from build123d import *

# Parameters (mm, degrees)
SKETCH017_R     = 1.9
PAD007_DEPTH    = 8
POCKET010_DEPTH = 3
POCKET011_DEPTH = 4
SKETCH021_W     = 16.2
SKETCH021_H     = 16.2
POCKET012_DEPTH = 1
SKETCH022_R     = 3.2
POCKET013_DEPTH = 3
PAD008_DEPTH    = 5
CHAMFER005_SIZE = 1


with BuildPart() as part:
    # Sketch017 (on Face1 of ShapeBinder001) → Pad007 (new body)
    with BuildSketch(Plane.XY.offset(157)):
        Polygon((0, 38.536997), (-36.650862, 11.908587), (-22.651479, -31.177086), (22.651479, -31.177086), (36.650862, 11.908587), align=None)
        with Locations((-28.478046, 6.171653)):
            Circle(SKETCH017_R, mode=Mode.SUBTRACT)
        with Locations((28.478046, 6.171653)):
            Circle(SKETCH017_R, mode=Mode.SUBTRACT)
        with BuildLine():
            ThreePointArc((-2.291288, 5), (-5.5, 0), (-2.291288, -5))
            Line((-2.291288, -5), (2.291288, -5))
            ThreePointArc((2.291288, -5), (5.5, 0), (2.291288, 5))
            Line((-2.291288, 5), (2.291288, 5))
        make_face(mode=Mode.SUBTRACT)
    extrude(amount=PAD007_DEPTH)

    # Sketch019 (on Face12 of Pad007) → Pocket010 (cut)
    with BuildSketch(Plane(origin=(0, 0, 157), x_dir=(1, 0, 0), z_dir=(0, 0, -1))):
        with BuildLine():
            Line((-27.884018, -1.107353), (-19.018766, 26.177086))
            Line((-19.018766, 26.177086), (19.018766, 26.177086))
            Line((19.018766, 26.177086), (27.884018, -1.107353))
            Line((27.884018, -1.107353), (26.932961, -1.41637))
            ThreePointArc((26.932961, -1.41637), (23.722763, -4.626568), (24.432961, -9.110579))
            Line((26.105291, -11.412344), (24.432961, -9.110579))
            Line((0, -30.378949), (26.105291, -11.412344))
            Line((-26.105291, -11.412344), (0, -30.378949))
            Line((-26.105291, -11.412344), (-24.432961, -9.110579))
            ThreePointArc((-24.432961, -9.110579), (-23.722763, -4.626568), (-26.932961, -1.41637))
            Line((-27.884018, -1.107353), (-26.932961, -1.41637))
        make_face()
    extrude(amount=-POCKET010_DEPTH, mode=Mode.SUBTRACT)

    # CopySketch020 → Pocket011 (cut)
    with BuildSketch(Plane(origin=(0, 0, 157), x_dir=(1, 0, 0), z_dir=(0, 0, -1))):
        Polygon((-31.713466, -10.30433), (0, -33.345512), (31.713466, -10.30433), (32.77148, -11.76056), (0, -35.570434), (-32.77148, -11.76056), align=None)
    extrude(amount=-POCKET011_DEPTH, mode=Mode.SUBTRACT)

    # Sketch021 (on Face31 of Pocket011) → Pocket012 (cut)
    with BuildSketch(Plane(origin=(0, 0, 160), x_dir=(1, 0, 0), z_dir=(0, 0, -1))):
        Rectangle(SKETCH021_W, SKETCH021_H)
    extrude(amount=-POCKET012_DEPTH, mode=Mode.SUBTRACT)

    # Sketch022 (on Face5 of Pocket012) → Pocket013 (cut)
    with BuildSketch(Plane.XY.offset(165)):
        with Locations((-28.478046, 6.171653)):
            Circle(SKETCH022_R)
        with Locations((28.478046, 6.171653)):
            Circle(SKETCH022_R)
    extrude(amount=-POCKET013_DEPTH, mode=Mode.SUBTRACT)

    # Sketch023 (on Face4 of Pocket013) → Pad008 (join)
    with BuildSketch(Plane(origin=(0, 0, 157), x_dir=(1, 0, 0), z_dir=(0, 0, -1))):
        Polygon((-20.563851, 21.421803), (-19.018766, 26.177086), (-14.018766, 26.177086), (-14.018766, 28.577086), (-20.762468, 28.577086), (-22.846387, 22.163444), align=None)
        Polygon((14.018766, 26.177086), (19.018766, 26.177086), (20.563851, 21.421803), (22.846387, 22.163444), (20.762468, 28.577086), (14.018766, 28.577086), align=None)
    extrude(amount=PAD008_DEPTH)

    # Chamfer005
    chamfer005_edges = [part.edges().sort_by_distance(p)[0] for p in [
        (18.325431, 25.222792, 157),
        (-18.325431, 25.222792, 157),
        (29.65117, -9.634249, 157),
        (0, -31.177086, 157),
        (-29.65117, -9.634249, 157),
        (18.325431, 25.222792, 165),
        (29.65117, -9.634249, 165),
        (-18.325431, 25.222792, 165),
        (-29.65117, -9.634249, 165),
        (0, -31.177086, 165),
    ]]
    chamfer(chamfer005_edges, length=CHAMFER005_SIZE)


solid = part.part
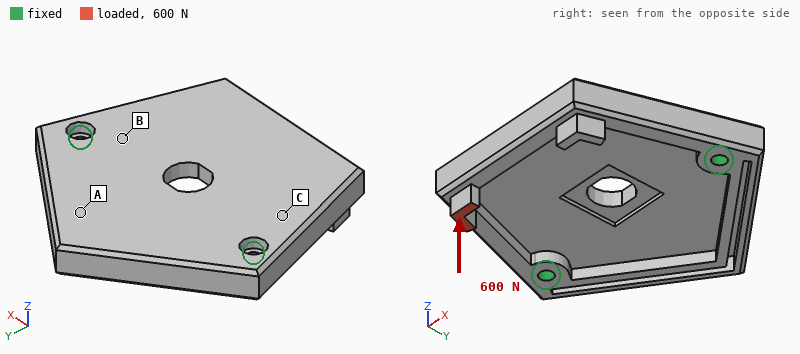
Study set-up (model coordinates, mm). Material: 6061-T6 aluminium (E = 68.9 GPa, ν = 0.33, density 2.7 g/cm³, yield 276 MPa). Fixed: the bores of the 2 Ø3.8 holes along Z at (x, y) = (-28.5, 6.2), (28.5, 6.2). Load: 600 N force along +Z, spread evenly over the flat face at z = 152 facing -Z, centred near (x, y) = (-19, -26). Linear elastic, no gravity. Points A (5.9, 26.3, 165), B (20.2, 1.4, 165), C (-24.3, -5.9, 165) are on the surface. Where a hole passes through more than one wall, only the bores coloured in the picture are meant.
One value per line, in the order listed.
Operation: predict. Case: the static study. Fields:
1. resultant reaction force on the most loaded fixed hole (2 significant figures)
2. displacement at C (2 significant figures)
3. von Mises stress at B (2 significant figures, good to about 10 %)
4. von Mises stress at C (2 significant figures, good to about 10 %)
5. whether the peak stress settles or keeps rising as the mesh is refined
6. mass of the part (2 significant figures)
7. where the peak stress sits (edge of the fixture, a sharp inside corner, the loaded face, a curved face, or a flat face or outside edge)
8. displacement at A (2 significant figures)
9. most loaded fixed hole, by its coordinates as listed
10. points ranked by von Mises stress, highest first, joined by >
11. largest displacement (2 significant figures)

630 N
0.062 mm
33 MPa
54 MPa
keeps rising
54 g
edge of the fixture
0.043 mm
(-28.5, 6.2)
C > B > A
0.27 mm
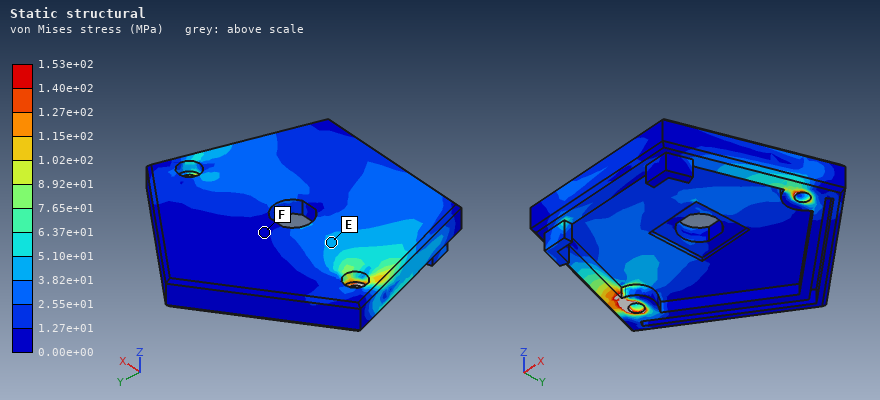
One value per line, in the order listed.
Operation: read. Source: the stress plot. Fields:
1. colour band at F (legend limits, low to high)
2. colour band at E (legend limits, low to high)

0.00e+00 to 1.27e+01 MPa
3.82e+01 to 5.10e+01 MPa
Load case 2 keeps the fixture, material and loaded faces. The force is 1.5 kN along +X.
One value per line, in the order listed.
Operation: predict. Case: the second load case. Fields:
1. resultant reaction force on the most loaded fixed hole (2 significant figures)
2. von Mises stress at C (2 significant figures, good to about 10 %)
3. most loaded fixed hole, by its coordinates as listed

1.3 kN
48 MPa
(-28.5, 6.2)
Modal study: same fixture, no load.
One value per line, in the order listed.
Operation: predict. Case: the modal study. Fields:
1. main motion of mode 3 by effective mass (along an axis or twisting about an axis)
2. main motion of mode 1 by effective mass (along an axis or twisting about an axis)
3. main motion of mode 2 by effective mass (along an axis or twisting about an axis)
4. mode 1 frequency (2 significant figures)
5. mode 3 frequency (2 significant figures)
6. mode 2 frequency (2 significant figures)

twisting about Y
along Z
along Z
2400 Hz
5800 Hz
4500 Hz
